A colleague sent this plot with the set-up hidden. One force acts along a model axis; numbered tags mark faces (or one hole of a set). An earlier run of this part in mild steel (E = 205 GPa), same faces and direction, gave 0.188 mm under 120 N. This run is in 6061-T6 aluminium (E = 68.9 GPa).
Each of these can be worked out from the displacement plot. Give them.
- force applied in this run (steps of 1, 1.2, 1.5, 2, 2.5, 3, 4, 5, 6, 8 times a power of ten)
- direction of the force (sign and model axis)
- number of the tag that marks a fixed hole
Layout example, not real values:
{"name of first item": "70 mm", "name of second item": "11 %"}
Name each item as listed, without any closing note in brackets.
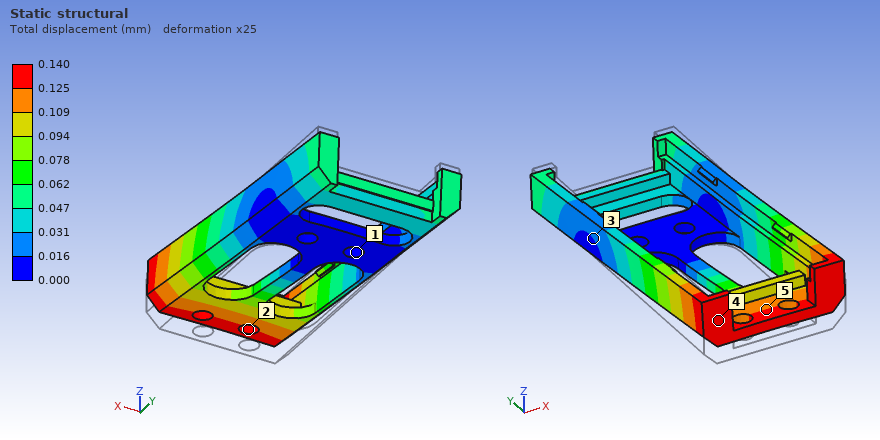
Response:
{"force applied in this run": "30 N", "direction of the force": "+Z", "number of the tag that marks a fixed hole": "1"}
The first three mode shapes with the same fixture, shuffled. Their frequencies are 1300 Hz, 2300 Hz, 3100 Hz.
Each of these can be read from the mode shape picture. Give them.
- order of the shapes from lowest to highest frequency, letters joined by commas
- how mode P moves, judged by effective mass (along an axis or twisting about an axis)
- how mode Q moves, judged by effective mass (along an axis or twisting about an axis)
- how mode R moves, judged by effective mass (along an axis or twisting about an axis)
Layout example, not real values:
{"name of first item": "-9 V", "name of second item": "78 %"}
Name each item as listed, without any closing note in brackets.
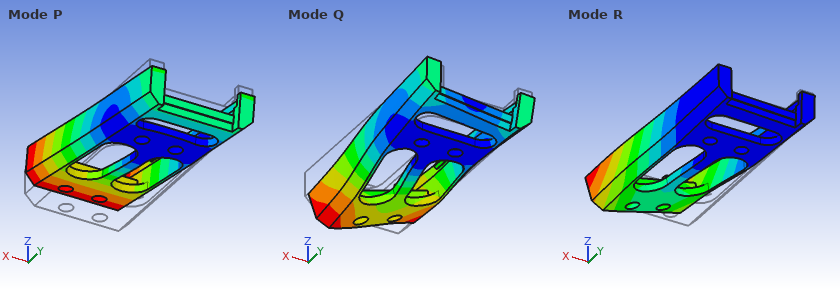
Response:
{"order of the shapes from lowest to highest frequency, letters joined by commas": "P, R, Q", "how mode P moves, judged by effective mass": "along Z", "how mode Q moves, judged by effective mass": "along X", "how mode R moves, judged by effective mass": "along X"}
